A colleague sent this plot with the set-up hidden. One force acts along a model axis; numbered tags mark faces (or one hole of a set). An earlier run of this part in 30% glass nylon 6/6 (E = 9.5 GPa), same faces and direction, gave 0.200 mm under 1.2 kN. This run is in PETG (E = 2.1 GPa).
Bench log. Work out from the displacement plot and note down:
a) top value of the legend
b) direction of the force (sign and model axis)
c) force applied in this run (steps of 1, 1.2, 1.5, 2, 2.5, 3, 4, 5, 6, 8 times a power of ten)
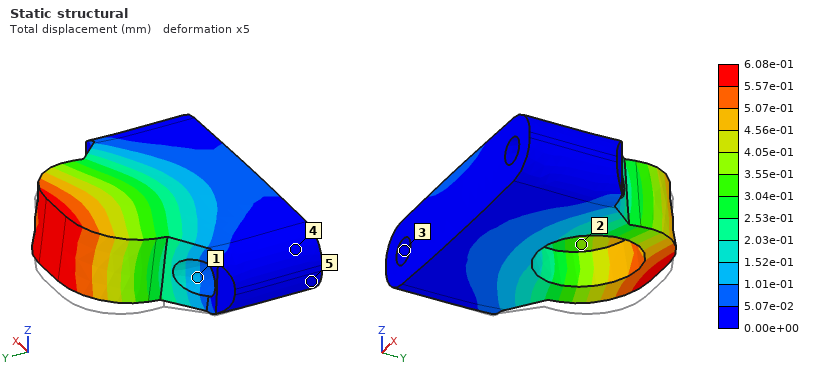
6.08e-01 mm
+Z
800 N
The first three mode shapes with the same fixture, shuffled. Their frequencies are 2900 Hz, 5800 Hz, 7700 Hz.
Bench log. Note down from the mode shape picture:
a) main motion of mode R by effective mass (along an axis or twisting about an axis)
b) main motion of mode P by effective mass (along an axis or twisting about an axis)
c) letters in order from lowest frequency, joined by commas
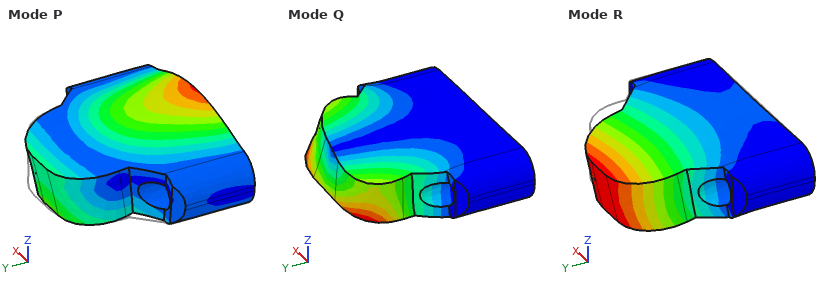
along Z
along Z
R, Q, P
